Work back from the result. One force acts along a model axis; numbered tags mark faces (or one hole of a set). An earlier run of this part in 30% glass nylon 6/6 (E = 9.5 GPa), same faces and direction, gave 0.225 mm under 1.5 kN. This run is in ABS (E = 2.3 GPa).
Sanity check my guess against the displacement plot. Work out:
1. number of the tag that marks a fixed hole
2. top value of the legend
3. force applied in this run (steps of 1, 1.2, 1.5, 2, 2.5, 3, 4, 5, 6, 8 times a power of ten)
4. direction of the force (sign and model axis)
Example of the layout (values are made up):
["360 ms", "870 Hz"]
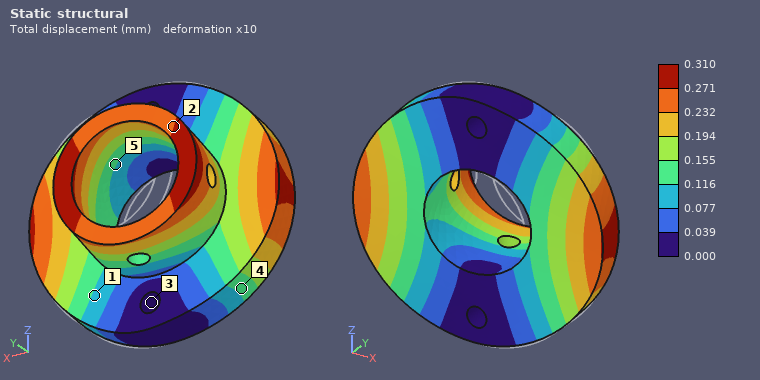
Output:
["3", "0.310 mm", "500 N", "-X"]
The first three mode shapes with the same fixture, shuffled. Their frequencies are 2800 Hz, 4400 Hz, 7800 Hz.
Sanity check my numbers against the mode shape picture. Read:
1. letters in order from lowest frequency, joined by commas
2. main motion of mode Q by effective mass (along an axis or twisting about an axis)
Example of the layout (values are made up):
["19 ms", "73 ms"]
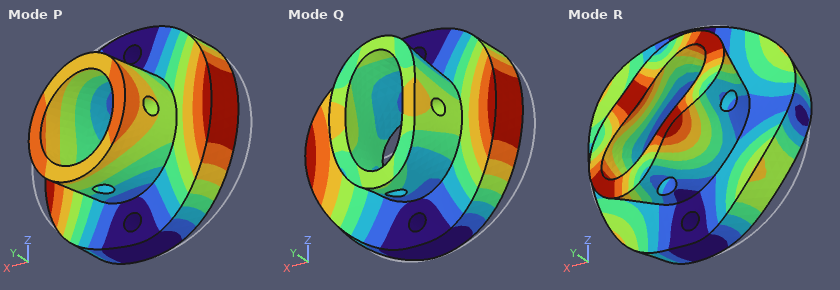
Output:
["P, Q, R", "along Y"]
